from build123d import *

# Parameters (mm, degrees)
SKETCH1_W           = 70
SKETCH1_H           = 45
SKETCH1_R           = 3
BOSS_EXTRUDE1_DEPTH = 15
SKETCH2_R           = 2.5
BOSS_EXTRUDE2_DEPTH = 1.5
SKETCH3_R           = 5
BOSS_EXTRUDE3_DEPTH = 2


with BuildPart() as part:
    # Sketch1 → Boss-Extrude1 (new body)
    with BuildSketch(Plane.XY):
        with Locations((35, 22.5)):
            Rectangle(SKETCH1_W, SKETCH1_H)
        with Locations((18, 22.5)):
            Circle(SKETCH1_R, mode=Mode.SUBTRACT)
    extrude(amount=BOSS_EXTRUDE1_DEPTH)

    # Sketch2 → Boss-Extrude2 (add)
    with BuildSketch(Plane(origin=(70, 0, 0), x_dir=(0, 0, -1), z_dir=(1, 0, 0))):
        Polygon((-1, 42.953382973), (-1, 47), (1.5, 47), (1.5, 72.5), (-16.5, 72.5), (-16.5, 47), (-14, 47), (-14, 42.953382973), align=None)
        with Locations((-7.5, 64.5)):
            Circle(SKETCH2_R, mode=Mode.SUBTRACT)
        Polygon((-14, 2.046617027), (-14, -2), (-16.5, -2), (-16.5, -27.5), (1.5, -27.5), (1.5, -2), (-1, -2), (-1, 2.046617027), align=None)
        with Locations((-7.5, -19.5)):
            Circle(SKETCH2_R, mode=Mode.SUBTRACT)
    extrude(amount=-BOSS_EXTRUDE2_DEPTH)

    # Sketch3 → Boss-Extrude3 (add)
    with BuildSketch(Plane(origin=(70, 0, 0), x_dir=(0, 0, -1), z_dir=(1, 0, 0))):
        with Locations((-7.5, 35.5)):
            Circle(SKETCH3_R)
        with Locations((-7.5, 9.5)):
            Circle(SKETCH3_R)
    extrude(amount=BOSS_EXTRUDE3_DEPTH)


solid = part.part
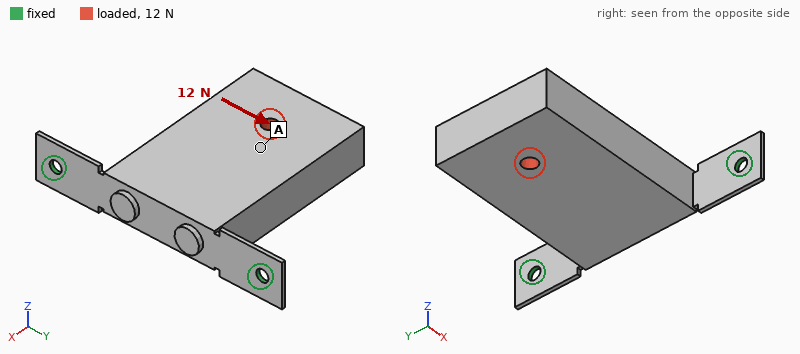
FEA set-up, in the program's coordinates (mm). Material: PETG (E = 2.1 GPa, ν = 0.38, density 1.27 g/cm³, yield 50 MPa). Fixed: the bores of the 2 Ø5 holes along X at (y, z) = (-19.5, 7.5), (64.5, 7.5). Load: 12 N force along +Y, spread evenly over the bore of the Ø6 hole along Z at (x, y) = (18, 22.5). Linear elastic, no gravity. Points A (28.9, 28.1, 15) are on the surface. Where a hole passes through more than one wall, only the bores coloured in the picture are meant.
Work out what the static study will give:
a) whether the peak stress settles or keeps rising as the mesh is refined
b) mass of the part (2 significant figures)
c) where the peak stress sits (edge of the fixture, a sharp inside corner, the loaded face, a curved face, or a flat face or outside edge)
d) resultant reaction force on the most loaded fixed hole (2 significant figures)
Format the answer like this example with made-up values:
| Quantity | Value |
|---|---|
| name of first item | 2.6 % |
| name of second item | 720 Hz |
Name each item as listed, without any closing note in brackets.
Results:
| Quantity | Value |
|---|---|
| whether the peak stress settles or keeps rising as the mesh is refined | keeps rising |
| mass of the part | 62 g |
| where the peak stress sits | edge of the fixture |
| resultant reaction force on the most loaded fixed hole | 11 N |
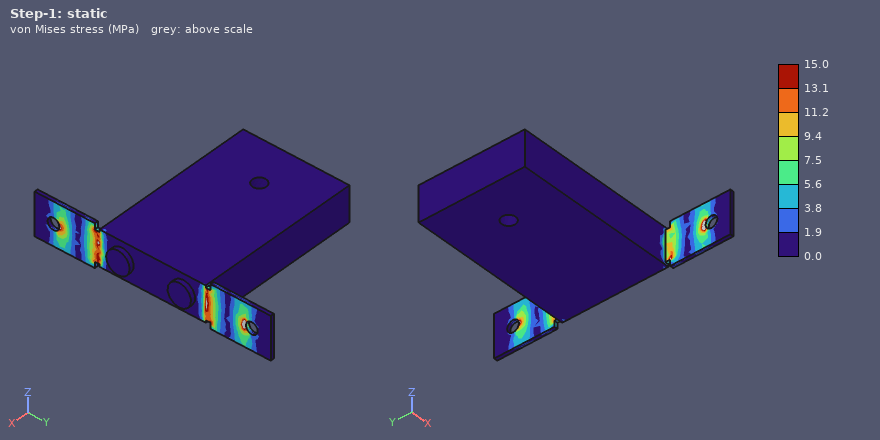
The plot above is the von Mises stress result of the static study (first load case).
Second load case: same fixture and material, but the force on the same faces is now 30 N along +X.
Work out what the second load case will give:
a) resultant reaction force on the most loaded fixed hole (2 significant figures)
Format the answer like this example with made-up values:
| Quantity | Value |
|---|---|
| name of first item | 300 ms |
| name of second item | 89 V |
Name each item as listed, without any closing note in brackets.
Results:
| Quantity | Value |
|---|---|
| resultant reaction force on the most loaded fixed hole | 18 N |
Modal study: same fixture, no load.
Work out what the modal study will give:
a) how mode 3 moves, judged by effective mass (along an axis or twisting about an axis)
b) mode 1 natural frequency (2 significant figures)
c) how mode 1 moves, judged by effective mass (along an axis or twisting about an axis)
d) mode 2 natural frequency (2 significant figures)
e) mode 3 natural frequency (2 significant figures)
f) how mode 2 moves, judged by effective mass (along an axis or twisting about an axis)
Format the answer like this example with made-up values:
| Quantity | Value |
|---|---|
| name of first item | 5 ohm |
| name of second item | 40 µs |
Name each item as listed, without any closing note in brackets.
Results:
| Quantity | Value |
|---|---|
| how mode 3 moves, judged by effective mass | along X |
| mode 1 natural frequency | 23 Hz |
| how mode 1 moves, judged by effective mass | along Z |
| mode 2 natural frequency | 92 Hz |
| mode 3 natural frequency | 120 Hz |
| how mode 2 moves, judged by effective mass | along Y |
